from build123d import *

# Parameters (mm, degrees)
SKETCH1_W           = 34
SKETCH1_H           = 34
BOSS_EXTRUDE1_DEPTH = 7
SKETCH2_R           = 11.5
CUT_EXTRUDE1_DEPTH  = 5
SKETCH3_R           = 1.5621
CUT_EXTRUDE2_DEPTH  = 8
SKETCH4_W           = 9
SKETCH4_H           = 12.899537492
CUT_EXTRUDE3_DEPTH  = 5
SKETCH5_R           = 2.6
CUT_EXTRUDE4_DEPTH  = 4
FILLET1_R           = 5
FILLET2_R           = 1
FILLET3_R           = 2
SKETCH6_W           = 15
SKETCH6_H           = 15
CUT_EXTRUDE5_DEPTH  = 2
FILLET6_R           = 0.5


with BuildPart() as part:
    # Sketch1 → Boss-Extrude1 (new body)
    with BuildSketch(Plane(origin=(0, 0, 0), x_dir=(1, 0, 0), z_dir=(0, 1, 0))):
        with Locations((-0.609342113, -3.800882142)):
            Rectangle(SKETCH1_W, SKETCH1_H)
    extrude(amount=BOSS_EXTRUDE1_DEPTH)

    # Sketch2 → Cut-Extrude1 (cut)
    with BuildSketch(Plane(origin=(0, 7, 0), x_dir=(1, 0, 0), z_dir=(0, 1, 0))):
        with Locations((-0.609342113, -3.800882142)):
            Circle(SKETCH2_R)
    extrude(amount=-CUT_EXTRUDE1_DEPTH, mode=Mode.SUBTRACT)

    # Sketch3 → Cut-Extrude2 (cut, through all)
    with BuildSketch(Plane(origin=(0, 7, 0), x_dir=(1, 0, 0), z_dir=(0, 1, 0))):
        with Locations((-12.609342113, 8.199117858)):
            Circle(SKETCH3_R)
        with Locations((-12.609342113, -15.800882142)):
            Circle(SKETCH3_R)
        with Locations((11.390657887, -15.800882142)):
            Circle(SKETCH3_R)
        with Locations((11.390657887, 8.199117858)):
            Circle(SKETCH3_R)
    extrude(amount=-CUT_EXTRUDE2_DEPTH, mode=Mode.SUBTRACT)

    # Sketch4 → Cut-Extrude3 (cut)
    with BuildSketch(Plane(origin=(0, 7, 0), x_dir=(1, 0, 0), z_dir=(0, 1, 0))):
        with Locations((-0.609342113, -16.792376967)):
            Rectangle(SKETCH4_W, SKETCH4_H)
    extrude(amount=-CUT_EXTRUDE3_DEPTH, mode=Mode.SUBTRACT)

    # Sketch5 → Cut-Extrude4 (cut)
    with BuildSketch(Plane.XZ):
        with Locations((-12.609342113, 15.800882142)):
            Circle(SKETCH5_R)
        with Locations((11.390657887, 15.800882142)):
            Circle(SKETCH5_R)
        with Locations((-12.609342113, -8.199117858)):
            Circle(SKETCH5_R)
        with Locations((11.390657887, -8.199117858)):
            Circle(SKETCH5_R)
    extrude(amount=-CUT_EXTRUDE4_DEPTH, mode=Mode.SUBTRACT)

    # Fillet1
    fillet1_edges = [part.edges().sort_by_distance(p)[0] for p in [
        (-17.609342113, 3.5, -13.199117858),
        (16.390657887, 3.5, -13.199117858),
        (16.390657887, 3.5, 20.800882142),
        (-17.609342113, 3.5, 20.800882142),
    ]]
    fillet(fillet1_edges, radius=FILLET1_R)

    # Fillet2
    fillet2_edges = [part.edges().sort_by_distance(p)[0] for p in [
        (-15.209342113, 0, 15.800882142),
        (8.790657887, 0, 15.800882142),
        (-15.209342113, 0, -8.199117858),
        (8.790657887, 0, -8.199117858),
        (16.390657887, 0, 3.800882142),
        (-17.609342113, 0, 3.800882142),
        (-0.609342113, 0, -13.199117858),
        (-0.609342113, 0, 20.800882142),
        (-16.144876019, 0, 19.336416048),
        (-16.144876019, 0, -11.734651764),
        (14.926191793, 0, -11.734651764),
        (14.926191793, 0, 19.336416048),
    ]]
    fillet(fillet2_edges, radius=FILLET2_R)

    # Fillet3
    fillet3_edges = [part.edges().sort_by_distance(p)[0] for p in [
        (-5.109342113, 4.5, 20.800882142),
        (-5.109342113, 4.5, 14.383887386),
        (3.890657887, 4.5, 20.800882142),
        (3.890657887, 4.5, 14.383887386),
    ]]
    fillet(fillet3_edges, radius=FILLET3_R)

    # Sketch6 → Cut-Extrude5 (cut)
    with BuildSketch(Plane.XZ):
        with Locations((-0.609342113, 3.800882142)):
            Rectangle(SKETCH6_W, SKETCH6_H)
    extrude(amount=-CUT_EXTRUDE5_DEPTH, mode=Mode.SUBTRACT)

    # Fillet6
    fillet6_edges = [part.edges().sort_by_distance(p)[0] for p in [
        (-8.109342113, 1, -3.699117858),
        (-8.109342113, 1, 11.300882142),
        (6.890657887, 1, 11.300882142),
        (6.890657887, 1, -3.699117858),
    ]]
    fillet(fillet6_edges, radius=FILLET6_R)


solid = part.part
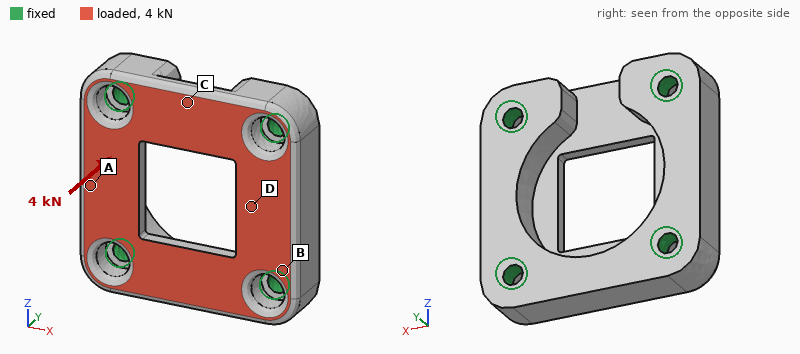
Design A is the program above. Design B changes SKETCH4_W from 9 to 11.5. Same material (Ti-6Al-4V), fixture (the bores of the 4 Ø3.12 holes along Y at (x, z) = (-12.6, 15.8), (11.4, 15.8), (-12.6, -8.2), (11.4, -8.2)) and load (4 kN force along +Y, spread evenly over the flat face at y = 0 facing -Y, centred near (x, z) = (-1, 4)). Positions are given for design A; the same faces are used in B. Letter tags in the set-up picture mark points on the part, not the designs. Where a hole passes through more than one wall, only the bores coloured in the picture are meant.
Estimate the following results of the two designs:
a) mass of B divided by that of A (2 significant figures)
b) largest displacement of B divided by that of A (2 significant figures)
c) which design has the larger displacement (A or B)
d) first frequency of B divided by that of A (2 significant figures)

0.98
1.2
B
1.0
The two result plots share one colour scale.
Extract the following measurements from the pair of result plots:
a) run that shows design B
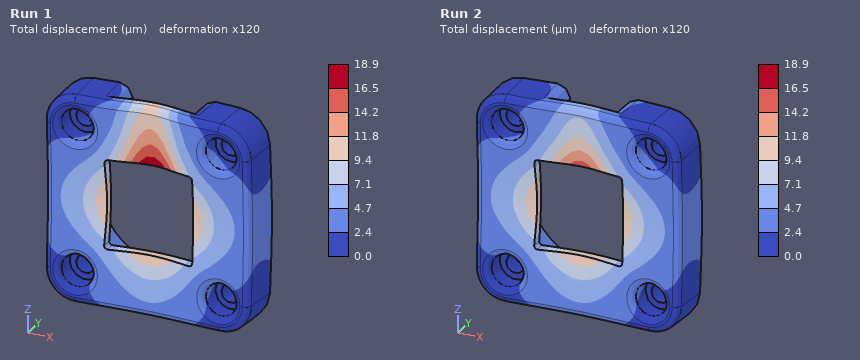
Run 1
